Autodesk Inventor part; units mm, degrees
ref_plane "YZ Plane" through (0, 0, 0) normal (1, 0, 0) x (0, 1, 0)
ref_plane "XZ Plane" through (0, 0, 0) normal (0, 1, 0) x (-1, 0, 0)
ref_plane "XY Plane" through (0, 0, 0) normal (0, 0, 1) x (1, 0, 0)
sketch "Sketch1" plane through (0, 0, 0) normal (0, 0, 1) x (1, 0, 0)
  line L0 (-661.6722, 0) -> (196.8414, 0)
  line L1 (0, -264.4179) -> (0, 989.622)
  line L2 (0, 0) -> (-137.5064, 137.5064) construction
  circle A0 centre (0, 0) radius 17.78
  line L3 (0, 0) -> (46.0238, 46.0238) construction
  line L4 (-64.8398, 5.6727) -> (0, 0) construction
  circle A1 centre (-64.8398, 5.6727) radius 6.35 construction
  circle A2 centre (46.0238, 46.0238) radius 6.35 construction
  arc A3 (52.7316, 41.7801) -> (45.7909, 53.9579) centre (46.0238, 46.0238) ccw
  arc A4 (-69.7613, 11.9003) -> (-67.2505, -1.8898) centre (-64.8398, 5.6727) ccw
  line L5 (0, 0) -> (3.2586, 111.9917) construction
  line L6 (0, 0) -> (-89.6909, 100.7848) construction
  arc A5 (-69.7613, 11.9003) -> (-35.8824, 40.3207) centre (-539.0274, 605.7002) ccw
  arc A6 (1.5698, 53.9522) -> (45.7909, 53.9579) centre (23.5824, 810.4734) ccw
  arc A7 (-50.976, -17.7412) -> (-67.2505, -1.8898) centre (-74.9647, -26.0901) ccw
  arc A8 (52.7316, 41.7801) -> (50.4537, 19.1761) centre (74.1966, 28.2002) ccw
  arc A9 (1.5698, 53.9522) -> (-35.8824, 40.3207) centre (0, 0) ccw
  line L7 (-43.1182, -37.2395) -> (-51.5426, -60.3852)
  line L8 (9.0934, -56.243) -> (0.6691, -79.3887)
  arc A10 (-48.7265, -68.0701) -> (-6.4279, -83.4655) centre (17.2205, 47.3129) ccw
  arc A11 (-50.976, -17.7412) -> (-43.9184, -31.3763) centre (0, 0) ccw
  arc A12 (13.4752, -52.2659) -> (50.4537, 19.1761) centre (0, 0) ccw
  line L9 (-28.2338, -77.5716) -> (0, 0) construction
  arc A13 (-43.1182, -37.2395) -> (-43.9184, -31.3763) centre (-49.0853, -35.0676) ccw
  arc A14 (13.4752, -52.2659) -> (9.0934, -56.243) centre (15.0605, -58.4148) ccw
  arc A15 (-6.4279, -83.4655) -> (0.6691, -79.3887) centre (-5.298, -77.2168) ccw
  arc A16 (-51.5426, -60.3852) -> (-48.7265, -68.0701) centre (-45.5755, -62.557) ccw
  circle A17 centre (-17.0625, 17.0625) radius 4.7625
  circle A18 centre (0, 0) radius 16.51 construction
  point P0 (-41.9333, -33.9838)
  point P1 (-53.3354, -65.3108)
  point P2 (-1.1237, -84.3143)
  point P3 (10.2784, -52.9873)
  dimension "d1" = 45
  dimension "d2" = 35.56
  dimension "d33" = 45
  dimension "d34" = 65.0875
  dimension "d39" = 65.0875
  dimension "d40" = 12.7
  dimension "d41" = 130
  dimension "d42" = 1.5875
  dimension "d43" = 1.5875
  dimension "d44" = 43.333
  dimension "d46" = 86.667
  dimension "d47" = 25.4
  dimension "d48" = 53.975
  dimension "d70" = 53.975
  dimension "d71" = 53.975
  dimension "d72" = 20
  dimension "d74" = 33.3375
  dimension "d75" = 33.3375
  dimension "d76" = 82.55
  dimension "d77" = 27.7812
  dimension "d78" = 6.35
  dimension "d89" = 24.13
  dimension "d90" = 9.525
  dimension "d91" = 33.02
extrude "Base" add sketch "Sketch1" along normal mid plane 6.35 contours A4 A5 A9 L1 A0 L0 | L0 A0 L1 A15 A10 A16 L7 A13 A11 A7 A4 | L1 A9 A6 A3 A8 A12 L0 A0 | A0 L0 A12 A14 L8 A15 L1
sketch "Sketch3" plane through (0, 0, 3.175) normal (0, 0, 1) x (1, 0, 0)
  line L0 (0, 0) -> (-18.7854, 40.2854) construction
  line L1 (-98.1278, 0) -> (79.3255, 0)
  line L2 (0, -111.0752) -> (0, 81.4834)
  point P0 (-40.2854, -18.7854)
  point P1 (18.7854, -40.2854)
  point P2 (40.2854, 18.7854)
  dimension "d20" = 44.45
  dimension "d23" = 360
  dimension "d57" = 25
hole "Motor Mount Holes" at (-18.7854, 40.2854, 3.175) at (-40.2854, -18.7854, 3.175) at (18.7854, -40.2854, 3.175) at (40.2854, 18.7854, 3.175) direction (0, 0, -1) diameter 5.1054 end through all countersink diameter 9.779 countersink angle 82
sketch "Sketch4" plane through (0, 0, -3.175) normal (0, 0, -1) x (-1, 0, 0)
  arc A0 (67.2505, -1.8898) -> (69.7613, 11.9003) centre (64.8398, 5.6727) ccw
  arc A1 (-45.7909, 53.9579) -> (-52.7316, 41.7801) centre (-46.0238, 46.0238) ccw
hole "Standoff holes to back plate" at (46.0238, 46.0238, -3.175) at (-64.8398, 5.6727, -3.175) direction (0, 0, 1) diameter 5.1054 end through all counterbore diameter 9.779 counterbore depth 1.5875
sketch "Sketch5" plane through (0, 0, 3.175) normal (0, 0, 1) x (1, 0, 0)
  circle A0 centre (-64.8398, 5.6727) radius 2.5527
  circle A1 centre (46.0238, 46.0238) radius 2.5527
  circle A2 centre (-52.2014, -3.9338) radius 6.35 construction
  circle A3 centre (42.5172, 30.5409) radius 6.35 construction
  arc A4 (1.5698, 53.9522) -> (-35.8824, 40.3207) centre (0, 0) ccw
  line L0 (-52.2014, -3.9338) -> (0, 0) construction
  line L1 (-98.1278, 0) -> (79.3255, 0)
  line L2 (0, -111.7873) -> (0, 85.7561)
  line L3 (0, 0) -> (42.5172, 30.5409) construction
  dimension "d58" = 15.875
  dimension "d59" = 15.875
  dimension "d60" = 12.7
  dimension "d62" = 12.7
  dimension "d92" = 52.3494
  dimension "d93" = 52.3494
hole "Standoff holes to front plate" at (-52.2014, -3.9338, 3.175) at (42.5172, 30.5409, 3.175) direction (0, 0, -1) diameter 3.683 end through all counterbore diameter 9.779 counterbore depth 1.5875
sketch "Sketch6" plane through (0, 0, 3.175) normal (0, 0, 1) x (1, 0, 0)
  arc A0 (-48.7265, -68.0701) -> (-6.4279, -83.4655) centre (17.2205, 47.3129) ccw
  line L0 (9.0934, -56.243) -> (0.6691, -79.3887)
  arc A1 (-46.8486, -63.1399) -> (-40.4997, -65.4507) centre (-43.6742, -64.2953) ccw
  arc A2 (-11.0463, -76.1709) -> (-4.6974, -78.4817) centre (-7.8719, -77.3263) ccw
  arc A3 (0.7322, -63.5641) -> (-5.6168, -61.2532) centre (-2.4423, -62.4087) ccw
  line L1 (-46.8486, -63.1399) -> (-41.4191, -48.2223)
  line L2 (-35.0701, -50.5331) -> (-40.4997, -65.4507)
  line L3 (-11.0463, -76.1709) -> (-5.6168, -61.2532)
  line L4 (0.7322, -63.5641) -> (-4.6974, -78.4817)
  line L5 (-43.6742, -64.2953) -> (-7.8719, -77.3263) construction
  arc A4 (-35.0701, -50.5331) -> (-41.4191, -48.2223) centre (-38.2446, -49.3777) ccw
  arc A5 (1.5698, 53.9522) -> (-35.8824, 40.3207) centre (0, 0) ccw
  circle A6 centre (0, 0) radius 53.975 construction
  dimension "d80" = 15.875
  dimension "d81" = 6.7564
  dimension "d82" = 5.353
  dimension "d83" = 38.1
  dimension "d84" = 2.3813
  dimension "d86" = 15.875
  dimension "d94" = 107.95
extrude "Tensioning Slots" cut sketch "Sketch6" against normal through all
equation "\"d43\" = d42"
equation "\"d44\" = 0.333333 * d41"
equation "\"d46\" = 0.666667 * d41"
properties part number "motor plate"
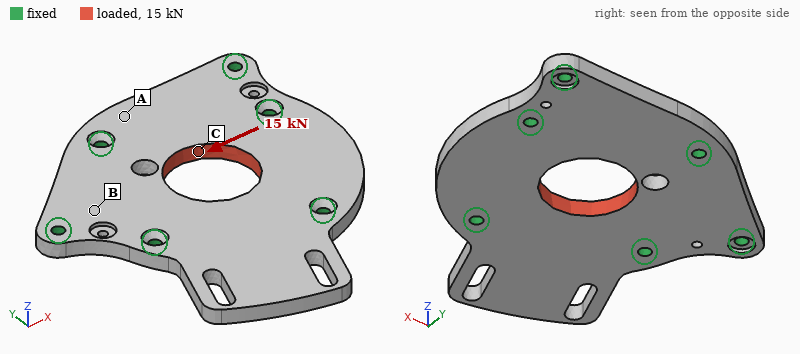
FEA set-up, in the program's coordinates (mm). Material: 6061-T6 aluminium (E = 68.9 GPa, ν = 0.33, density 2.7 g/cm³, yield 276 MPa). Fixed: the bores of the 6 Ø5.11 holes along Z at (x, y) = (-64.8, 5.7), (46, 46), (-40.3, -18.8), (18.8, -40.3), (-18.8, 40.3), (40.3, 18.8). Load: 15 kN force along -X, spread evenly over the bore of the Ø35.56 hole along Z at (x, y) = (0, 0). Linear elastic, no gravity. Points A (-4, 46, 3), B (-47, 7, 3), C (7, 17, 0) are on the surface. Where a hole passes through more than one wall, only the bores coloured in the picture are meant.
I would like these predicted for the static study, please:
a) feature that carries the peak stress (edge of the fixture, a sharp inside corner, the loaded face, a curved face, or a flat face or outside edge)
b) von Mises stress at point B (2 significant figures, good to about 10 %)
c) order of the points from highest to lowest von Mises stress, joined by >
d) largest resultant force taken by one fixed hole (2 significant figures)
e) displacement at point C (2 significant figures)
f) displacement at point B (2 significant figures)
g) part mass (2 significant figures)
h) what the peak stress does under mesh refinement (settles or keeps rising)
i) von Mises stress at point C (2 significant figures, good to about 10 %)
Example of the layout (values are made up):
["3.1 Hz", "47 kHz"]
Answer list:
["edge of the fixture", "20 MPa", "C > B > A", "3.6 kN", "13 µm", "5.6 µm", "170 g", "keeps rising", "35 MPa"]
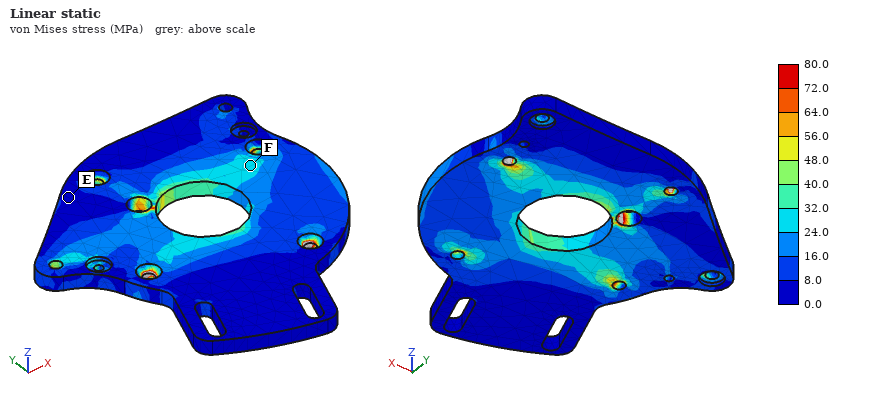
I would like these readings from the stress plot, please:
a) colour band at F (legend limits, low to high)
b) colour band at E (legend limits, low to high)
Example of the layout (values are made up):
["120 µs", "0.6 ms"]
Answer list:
["24.0 to 32.0 MPa", "0.0 to 8.0 MPa"]
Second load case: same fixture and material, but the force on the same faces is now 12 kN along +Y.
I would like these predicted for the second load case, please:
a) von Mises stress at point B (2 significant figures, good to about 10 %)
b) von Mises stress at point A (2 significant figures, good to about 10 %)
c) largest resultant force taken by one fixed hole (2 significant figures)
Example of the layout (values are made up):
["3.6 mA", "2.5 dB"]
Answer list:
["7.3 MPa", "7.8 MPa", "3.3 kN"]
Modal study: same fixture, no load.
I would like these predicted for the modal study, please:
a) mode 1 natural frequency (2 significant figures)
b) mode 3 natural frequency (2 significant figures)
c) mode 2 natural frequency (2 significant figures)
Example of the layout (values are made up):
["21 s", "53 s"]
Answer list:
["1800 Hz", "5500 Hz", "5000 Hz"]
